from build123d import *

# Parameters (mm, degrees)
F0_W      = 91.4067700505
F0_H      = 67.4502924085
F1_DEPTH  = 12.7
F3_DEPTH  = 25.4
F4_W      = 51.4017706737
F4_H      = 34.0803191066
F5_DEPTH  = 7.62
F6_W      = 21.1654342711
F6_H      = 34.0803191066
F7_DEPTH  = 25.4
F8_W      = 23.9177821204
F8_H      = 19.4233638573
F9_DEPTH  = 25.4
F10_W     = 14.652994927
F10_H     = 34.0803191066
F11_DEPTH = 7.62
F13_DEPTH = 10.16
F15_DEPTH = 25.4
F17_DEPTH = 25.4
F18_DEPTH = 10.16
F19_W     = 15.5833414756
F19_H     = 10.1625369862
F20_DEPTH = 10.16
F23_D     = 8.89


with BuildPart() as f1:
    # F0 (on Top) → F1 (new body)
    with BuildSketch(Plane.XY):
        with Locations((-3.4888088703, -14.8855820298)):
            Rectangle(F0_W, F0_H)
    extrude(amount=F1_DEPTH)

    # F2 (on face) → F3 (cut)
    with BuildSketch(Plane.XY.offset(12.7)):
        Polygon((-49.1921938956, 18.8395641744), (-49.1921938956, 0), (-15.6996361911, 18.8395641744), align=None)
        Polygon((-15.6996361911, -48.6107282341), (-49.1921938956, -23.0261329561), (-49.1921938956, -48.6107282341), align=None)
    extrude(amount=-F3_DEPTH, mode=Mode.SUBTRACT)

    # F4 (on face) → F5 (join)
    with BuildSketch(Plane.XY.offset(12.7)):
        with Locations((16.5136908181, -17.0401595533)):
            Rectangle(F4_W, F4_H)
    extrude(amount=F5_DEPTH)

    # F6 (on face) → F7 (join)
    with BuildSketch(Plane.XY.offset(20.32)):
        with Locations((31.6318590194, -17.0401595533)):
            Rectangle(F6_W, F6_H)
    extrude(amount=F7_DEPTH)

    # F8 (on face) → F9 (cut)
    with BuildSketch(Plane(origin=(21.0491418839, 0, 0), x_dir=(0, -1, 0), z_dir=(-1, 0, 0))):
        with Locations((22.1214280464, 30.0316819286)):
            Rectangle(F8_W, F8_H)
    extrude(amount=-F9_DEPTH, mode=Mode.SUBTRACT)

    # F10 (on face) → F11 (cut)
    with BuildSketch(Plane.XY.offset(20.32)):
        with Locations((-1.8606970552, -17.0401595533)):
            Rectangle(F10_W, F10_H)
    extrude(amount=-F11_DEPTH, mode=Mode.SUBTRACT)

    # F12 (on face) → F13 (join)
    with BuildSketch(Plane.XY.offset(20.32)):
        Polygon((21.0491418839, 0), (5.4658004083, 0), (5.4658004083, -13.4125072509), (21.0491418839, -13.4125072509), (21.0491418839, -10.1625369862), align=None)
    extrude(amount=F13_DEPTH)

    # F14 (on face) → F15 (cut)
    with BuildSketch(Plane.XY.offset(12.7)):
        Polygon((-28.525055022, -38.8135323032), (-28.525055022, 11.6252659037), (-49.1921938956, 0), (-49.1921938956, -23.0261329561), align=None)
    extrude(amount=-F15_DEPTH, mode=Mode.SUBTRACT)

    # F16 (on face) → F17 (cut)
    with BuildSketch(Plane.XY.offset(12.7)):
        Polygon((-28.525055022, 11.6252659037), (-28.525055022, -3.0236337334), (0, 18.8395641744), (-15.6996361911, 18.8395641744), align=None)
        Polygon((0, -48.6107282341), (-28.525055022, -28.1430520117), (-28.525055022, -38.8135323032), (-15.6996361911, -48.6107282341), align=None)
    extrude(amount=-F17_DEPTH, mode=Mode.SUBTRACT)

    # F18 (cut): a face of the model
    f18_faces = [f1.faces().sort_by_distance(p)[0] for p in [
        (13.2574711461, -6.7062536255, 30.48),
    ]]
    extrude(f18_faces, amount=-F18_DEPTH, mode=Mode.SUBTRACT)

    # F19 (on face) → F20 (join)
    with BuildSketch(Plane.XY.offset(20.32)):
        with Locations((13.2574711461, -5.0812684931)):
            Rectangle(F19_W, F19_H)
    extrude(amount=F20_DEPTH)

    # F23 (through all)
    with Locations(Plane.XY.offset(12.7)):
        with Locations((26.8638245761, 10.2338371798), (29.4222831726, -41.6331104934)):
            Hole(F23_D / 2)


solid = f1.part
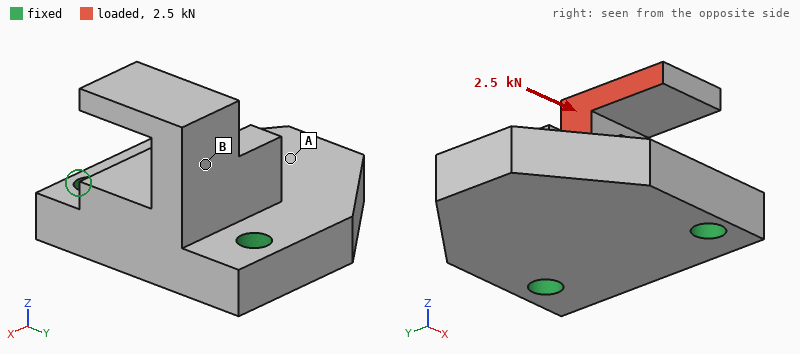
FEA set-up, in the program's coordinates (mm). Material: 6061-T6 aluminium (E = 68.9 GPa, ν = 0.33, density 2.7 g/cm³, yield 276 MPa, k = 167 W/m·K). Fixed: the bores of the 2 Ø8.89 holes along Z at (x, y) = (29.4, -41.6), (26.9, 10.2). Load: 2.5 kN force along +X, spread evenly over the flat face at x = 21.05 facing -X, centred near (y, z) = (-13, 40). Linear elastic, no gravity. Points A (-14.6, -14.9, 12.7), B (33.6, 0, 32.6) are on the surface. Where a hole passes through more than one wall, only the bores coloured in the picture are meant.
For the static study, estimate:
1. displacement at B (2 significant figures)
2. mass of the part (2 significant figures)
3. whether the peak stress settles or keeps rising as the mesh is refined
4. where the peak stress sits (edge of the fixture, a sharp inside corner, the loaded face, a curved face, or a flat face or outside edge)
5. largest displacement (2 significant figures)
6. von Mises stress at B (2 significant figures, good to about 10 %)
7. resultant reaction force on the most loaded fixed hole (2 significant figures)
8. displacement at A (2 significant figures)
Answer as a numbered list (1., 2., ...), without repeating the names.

1. 0.035 mm
2. 190 g
3. keeps rising
4. edge of the fixture
5. 0.17 mm
6. 31 MPa
7. 1.4 kN
8. 0.039 mm
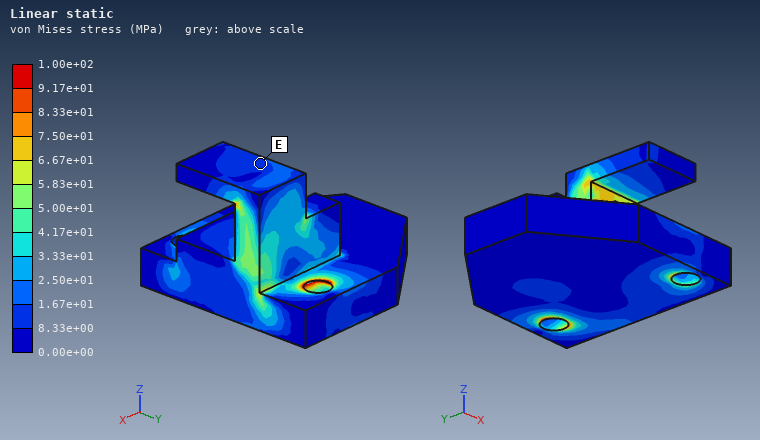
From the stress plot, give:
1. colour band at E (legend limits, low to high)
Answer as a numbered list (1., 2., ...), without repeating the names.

1. 8.33e+00 to 1.67e+01 MPa
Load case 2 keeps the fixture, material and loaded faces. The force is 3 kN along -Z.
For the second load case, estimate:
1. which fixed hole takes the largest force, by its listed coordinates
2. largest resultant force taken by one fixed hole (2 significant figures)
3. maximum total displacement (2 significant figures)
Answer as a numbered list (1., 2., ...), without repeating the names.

1. (26.9, 10.2)
2. 1.8 kN
3. 0.35 mm
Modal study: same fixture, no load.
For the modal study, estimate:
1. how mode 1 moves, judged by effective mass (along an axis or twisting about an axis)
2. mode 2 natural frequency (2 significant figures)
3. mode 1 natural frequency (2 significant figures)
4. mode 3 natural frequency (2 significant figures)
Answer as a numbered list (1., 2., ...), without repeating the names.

1. along Z
2. 4300 Hz
3. 3800 Hz
4. 6300 Hz
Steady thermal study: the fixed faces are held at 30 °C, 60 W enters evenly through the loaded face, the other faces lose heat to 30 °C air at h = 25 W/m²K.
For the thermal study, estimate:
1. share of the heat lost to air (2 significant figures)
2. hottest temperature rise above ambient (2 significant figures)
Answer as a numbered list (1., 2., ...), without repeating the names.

1. 7.0 %
2. 68 K
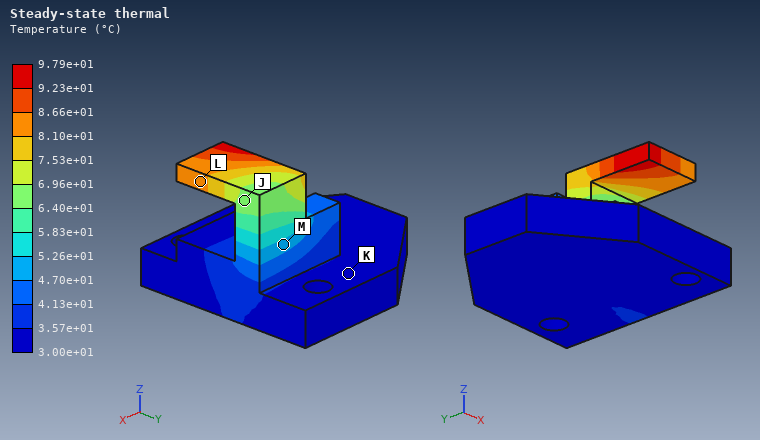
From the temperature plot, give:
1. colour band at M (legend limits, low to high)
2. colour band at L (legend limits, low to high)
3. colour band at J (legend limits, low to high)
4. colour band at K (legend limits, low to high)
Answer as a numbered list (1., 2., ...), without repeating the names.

1. 4.70e+01 to 5.26e+01 °C
2. 8.10e+01 to 8.66e+01 °C
3. 6.40e+01 to 6.96e+01 °C
4. 3.00e+01 to 3.57e+01 °C
